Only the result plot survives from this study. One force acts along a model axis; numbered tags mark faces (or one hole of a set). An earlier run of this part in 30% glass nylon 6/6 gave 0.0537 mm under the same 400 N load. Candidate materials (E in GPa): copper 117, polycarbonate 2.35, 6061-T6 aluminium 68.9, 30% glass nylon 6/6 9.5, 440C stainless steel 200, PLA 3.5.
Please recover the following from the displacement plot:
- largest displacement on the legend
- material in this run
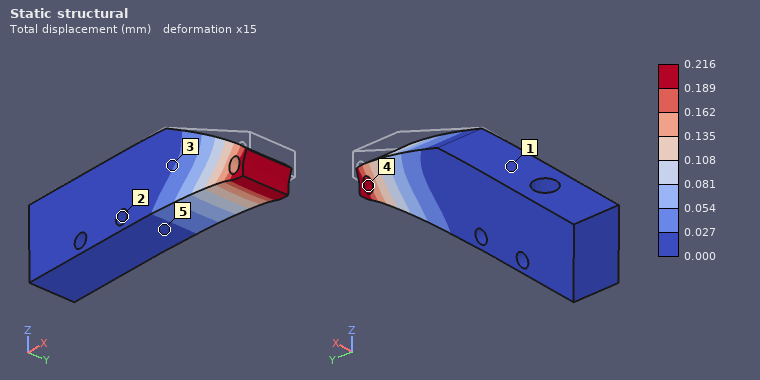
0.216 mm
polycarbonate
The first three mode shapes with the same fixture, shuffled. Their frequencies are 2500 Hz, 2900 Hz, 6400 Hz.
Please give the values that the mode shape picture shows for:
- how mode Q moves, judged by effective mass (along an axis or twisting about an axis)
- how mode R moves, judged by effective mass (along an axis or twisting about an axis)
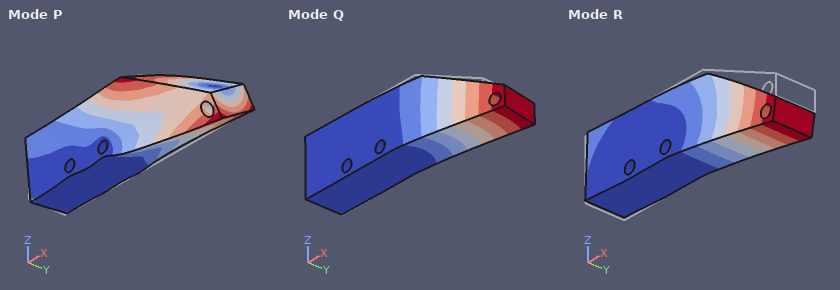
along Y
along Z
